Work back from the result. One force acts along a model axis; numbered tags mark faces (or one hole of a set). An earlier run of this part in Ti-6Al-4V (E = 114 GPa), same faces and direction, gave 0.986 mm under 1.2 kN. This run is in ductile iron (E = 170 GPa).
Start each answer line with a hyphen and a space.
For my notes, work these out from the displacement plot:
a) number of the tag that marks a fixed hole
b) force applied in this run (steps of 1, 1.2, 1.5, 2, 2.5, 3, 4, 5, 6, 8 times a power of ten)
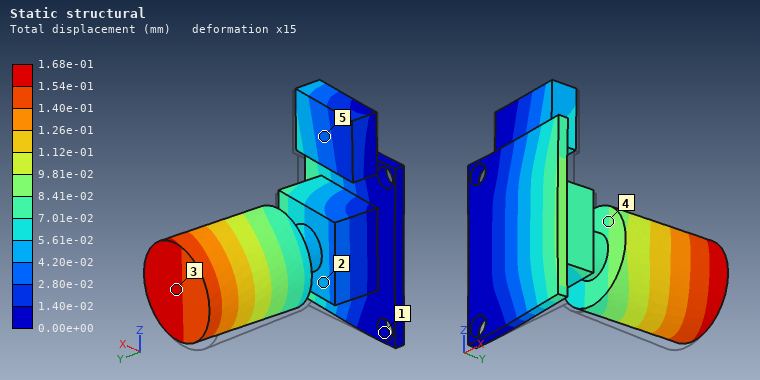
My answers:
- 1
- 300 N
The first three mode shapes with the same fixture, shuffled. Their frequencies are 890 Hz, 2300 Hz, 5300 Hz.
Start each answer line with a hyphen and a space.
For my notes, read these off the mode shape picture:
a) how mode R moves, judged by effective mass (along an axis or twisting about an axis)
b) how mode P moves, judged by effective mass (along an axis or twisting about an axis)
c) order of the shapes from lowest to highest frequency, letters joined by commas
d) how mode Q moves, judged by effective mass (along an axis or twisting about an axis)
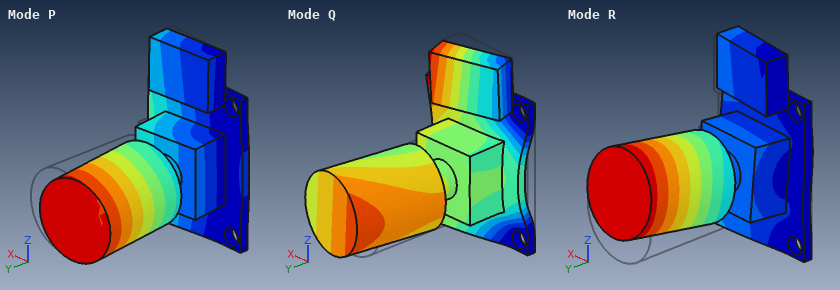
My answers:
- along Z
- along X
- P, R, Q
- along Y
